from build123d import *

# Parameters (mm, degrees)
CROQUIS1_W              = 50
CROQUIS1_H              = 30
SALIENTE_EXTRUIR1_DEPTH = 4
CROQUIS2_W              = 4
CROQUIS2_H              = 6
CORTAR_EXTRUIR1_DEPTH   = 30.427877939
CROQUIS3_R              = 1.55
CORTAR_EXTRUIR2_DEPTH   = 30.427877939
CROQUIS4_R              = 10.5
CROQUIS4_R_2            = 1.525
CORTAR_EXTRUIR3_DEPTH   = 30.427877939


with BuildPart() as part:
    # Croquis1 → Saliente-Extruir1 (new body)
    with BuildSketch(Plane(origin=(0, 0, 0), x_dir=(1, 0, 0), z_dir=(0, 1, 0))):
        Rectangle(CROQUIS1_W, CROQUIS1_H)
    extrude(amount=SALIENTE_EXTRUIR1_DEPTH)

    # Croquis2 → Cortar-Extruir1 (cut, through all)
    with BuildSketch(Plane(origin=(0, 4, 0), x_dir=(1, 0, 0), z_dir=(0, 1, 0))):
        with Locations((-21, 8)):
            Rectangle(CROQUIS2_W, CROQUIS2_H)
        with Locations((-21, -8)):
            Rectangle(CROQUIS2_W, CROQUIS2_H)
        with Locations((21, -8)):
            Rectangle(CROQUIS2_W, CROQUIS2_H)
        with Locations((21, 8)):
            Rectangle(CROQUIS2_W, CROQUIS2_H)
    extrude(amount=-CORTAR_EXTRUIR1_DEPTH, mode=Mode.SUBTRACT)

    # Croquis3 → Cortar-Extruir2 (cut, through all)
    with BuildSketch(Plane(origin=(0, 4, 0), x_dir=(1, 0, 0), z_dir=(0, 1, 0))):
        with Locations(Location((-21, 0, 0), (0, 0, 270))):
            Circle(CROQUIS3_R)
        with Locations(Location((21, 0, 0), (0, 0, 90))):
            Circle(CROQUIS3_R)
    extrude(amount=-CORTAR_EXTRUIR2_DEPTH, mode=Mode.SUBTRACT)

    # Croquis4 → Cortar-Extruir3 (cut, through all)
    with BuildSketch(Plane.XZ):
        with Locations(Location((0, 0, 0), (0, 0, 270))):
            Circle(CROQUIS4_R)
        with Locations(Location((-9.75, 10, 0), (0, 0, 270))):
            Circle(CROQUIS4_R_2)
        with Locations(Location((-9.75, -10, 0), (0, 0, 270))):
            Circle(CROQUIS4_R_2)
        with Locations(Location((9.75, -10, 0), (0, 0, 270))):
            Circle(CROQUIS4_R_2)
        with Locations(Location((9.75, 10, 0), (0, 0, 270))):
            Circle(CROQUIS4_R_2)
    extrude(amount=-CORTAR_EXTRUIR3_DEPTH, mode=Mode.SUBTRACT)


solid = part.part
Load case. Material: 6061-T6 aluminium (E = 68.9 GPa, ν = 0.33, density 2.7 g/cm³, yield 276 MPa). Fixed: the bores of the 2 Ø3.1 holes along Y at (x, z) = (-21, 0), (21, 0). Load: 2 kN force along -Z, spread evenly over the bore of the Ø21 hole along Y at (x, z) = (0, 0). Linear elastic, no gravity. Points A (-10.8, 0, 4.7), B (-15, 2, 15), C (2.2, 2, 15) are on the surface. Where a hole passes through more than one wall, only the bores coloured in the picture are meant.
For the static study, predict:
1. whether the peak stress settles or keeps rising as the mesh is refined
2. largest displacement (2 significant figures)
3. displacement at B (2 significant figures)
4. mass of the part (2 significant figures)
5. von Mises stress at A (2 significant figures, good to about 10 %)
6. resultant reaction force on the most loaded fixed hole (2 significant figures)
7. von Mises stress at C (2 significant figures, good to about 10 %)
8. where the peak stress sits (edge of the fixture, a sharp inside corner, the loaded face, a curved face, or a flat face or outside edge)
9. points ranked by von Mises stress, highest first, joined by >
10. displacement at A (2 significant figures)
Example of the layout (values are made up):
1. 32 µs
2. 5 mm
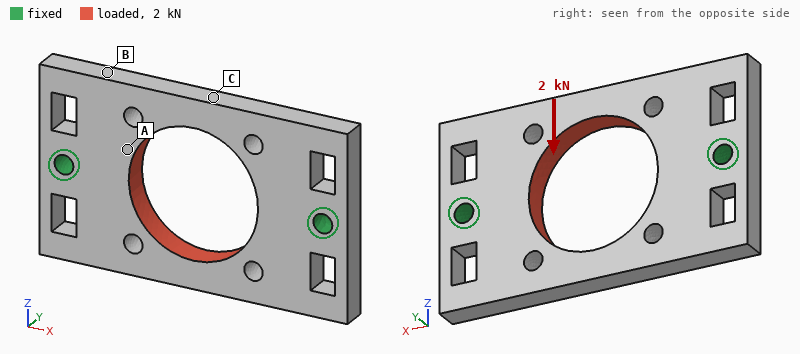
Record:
1. keeps rising
2. 15 µm
3. 7.7 µm
4. 11 g
5. 26 MPa
6. 1.0 kN
7. 43 MPa
8. edge of the fixture
9. C > A > B
10. 8.8 µm
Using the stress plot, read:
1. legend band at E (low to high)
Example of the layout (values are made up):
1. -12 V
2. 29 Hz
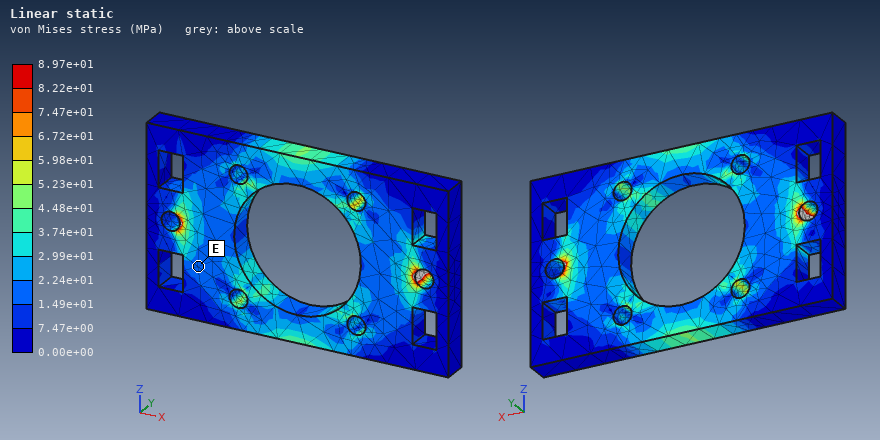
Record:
1. 1.49e+01 to 2.24e+01 MPa
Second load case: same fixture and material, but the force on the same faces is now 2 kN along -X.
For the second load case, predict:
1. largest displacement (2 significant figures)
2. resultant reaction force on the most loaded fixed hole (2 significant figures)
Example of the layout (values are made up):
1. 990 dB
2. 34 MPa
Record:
1. 8.8 µm
2. 1.0 kN
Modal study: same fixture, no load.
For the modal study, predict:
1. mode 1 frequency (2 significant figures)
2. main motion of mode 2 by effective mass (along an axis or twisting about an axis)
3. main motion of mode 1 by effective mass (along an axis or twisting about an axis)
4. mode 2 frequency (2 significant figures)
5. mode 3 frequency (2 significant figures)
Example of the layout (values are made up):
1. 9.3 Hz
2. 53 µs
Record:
1. 7100 Hz
2. along Y
3. twisting about X
4. 8600 Hz
5. 13 kHz
